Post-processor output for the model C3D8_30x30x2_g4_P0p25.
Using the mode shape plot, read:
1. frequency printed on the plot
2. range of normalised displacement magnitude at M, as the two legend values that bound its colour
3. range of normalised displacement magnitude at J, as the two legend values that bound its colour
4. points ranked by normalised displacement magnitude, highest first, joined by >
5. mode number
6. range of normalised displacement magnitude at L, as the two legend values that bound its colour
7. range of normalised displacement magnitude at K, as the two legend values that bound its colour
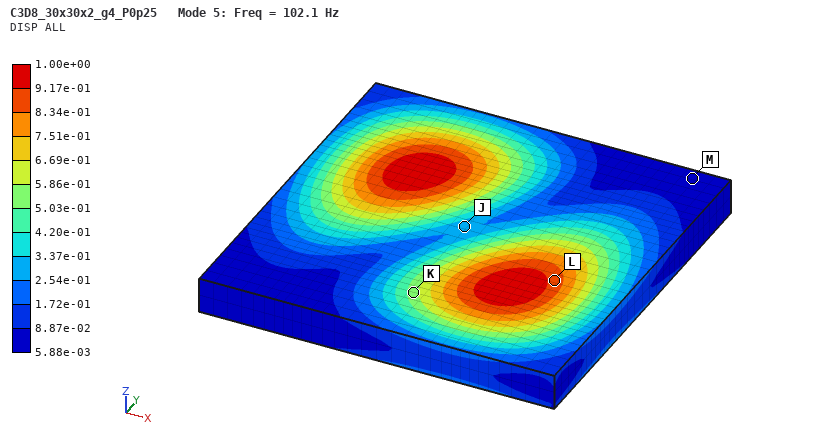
102.1 Hz
5.88e-03 to 8.87e-02
2.54e-01 to 3.37e-01
L > K > J > M
5
8.34e-01 to 9.17e-01
5.03e-01 to 5.86e-01
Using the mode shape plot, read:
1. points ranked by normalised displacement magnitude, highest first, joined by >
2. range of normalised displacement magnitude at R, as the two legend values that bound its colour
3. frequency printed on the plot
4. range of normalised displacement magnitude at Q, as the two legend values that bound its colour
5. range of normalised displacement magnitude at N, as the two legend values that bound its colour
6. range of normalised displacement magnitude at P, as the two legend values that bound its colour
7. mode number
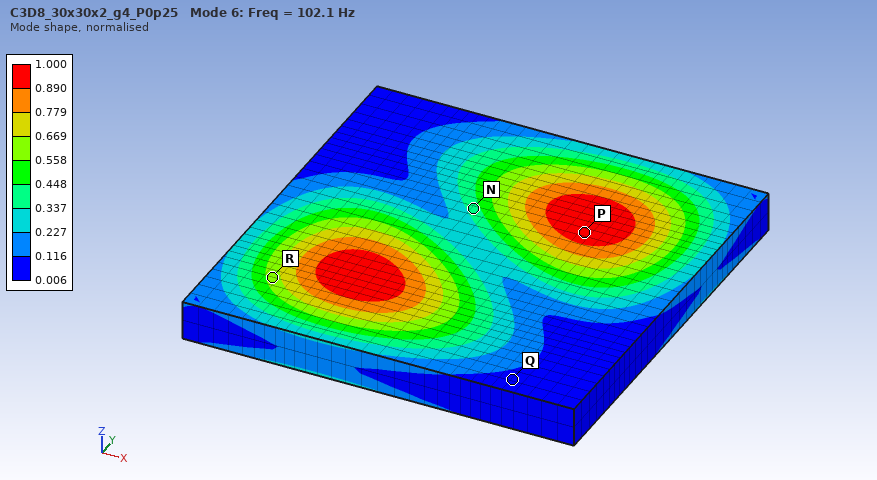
P > R > N > Q
0.558 to 0.669
102.1 Hz
0.006 to 0.116
0.337 to 0.448
0.890 to 1.000
6
